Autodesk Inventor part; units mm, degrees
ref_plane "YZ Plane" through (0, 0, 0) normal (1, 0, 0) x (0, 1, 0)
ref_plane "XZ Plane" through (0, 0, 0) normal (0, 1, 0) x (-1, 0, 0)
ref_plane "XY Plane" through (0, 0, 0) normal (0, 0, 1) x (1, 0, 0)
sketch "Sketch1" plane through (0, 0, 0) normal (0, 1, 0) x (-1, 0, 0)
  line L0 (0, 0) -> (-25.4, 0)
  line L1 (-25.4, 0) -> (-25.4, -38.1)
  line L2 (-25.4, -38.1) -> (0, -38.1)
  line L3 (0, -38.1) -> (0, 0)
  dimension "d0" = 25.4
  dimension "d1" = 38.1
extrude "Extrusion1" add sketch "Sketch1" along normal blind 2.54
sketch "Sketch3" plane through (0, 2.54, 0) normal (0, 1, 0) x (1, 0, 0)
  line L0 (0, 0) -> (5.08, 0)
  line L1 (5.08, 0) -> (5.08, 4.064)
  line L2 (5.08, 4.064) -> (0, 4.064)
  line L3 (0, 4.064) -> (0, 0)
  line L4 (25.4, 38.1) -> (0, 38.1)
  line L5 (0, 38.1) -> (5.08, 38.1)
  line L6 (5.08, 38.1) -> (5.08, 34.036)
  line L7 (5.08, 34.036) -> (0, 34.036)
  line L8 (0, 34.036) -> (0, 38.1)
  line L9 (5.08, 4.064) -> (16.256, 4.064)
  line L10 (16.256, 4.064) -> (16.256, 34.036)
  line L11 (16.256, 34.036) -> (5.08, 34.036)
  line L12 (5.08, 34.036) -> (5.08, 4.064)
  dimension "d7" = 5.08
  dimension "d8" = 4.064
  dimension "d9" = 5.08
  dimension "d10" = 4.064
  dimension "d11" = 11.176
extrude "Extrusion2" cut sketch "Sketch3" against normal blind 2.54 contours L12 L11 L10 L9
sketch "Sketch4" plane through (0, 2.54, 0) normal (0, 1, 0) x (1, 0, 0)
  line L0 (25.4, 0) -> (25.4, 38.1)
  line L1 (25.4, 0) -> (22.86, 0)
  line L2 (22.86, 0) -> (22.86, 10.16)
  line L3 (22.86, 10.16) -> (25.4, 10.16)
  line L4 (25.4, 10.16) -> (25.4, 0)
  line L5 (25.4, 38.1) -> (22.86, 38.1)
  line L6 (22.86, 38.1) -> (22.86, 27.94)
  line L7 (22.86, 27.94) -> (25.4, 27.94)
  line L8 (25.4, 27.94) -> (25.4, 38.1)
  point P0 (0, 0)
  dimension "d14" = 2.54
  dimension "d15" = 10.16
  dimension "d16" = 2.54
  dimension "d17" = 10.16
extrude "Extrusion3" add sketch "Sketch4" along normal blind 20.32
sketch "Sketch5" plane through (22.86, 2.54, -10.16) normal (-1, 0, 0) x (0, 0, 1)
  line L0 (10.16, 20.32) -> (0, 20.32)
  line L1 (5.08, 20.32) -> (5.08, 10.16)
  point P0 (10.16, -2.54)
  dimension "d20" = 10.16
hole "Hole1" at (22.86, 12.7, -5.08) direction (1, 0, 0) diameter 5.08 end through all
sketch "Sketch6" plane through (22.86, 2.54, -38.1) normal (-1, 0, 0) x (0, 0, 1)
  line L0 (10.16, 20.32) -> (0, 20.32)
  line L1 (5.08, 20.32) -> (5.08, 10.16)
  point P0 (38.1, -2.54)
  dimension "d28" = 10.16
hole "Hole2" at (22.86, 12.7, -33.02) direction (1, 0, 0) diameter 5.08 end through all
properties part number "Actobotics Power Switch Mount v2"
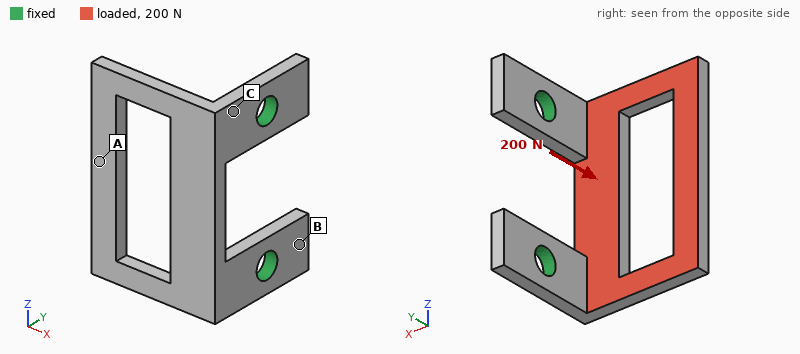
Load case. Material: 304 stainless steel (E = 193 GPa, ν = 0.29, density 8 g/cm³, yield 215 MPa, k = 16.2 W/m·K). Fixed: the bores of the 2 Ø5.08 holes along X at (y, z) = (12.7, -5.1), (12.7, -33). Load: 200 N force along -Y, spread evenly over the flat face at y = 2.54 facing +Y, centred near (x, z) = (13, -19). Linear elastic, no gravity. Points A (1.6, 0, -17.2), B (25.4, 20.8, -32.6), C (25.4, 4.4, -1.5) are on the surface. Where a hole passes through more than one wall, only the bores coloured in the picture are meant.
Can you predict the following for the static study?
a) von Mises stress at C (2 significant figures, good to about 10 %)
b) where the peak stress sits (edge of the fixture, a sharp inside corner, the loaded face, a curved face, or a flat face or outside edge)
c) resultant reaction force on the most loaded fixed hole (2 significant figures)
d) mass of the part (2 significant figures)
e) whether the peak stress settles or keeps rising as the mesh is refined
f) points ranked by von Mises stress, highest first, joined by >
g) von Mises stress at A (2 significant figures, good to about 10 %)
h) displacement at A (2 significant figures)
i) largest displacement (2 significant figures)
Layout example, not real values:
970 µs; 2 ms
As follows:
97 MPa; a sharp inside corner; 100 N; 20 g; keeps rising; C > A > B; 29 MPa; 0.18 mm; 0.20 mm
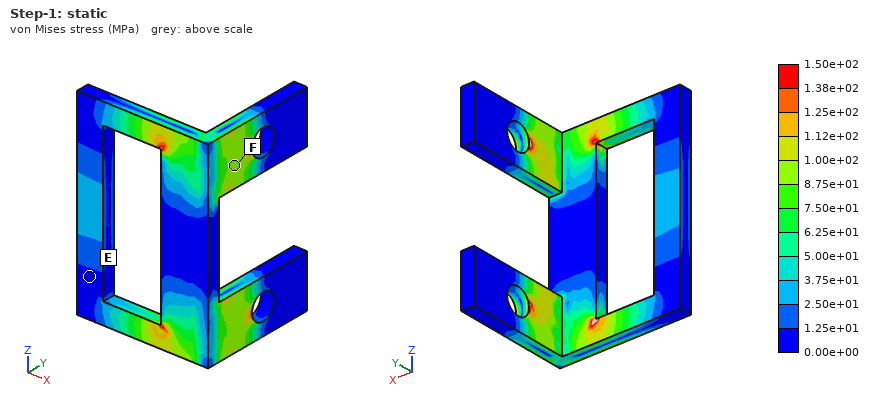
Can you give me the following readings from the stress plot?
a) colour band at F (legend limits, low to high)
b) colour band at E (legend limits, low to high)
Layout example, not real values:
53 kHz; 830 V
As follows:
8.75e+01 to 1.00e+02 MPa; 0.00e+00 to 1.25e+01 MPa
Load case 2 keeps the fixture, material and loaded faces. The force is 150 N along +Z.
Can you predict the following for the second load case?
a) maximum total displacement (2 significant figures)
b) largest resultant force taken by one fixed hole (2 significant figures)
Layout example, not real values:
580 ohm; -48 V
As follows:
20 µm; 90 N
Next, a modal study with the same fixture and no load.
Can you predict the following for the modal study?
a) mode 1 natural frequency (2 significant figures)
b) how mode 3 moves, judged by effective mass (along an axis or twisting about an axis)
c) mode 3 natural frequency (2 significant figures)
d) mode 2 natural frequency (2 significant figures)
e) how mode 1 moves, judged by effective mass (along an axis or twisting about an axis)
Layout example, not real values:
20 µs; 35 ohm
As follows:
1700 Hz; along Z; 5500 Hz; 3800 Hz; along Y
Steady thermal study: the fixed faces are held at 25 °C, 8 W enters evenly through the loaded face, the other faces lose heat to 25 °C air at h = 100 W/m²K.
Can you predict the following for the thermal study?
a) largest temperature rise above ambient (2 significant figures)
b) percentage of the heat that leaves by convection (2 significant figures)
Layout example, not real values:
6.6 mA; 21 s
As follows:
63 K; 73 %
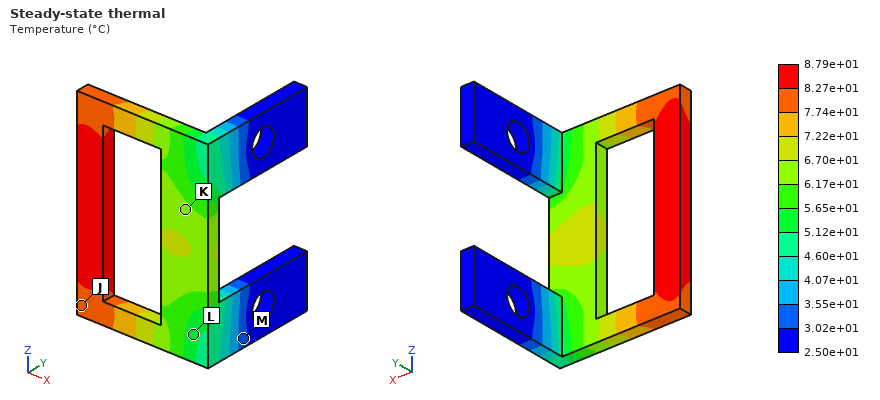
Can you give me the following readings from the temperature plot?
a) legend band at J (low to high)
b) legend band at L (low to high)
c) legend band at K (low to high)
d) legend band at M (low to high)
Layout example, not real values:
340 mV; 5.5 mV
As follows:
7.74e+01 to 8.27e+01 °C; 5.12e+01 to 5.65e+01 °C; 6.17e+01 to 6.70e+01 °C; 3.02e+01 to 3.55e+01 °C
